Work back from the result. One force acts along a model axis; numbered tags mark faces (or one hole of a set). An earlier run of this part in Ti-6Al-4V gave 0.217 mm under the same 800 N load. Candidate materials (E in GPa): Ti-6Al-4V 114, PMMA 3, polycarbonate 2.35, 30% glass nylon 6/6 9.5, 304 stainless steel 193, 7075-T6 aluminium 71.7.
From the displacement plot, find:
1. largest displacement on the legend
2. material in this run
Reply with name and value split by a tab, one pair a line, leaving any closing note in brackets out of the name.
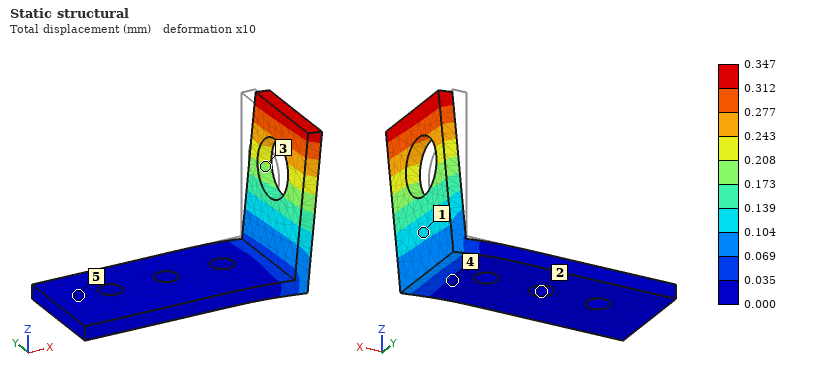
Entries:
largest displacement on the legend	0.347 mm
material in this run	7075-T6 aluminium
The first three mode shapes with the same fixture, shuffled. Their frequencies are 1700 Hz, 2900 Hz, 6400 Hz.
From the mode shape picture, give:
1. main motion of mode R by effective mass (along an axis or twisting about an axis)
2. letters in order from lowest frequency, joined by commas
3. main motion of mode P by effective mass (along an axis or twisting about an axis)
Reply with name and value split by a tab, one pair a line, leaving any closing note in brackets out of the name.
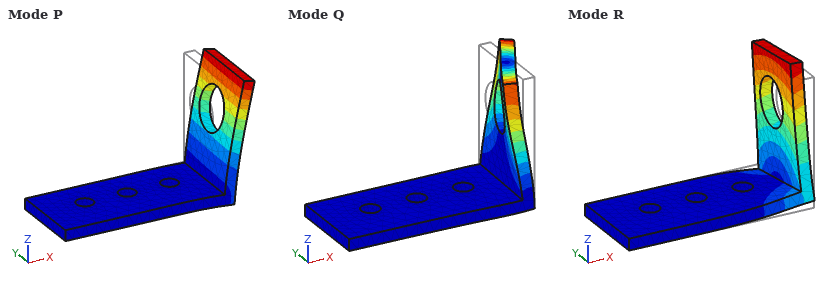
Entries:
main motion of mode R by effective mass	along Y
letters in order from lowest frequency, joined by commas	P, R, Q
main motion of mode P by effective mass	along X
